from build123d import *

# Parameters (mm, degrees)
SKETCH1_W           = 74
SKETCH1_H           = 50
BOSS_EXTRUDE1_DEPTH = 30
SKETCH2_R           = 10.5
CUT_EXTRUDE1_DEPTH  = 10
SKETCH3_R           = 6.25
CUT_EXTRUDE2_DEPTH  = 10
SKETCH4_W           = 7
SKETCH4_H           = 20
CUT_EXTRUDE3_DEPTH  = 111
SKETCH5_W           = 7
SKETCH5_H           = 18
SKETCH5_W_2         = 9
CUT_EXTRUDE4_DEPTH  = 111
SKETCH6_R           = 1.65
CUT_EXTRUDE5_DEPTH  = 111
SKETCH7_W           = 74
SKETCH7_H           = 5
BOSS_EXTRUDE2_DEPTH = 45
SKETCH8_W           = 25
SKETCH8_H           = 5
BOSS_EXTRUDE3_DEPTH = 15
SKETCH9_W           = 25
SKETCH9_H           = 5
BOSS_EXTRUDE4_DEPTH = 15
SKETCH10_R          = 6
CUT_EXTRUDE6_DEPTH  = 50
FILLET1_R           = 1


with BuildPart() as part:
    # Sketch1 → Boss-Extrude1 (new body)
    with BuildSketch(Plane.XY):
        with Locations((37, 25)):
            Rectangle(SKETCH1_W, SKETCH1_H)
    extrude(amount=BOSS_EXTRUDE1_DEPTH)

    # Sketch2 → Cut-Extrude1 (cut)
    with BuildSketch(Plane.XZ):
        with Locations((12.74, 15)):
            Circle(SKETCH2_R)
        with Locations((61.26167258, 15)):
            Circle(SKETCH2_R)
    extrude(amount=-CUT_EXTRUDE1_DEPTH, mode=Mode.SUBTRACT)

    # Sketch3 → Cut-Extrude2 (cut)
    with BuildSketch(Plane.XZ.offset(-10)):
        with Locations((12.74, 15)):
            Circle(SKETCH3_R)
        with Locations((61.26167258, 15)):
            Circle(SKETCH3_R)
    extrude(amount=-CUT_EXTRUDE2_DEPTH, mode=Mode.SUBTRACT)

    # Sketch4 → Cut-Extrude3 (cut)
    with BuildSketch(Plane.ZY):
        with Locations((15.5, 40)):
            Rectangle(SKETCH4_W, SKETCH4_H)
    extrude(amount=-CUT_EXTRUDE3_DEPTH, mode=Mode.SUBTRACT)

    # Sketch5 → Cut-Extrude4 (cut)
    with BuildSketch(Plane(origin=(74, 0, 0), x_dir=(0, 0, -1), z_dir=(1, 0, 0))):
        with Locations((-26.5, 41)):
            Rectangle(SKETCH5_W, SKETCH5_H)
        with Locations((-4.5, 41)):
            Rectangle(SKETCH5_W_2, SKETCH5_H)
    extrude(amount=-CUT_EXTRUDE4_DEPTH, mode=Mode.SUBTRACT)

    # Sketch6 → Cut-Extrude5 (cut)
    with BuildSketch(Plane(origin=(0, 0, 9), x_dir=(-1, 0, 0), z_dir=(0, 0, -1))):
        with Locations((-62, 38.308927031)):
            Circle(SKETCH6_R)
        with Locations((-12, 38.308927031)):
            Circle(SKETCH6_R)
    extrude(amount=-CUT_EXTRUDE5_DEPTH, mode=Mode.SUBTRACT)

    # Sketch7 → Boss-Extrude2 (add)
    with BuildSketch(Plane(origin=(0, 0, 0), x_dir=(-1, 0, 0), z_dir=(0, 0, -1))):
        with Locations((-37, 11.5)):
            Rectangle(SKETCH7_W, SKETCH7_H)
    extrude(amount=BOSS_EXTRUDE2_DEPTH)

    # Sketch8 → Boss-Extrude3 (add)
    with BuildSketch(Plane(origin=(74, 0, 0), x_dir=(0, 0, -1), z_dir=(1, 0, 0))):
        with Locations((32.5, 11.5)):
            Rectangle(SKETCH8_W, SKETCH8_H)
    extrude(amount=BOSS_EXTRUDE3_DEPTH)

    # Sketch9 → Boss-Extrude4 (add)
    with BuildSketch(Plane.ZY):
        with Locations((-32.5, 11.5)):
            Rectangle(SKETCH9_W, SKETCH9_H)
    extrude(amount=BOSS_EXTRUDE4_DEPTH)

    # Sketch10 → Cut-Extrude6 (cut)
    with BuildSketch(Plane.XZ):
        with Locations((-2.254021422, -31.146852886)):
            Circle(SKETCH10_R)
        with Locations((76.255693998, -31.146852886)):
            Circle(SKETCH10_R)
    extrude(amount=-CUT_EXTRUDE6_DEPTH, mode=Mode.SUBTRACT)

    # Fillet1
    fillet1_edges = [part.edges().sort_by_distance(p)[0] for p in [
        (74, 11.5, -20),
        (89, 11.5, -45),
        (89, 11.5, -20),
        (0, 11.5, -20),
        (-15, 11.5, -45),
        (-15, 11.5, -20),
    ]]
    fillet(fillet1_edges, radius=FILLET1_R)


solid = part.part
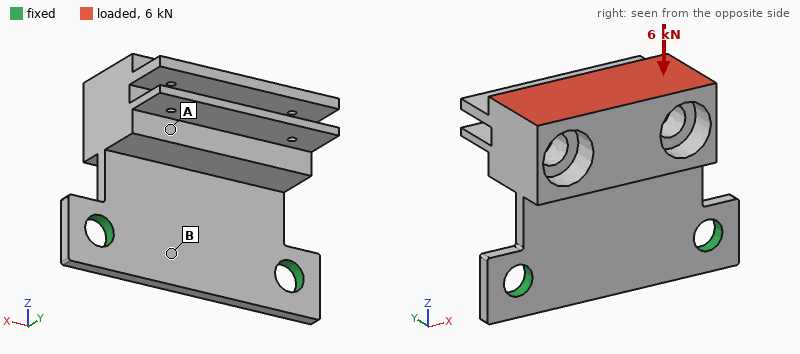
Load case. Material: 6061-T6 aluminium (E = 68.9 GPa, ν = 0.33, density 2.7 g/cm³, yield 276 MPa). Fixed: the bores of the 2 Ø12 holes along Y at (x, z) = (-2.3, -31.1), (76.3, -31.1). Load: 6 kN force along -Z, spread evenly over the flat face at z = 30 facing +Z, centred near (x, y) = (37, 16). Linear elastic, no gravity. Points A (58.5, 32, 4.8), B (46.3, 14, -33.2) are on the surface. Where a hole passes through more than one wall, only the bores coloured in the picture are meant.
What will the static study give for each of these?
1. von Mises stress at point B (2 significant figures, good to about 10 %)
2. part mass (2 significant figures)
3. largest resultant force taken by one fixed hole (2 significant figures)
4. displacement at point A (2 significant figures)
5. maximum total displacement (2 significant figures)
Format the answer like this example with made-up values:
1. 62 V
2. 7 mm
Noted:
1. 31 MPa
2. 240 g
3. 3.2 kN
4. 0.49 mm
5. 0.91 mm
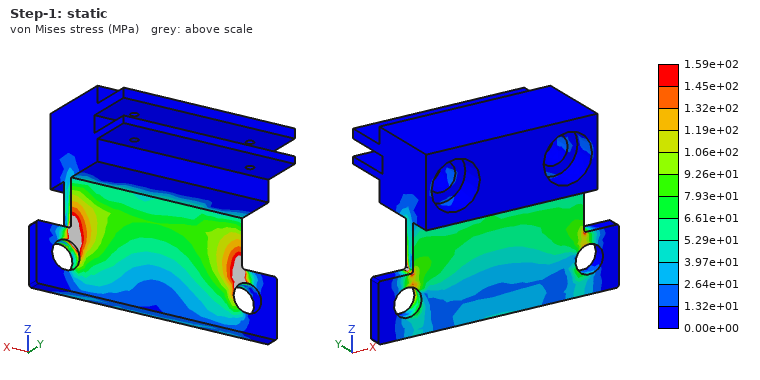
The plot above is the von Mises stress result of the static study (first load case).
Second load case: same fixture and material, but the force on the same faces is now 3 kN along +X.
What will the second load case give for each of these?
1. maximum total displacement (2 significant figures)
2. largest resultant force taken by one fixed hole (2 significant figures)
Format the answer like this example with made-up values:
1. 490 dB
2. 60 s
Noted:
1. 71 µm
2. 2.9 kN
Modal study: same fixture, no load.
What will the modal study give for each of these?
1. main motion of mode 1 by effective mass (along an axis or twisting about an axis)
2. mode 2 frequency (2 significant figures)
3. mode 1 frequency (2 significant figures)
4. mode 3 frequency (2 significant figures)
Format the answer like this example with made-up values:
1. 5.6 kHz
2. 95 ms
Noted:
1. along Y
2. 1600 Hz
3. 400 Hz
4. 2600 Hz
